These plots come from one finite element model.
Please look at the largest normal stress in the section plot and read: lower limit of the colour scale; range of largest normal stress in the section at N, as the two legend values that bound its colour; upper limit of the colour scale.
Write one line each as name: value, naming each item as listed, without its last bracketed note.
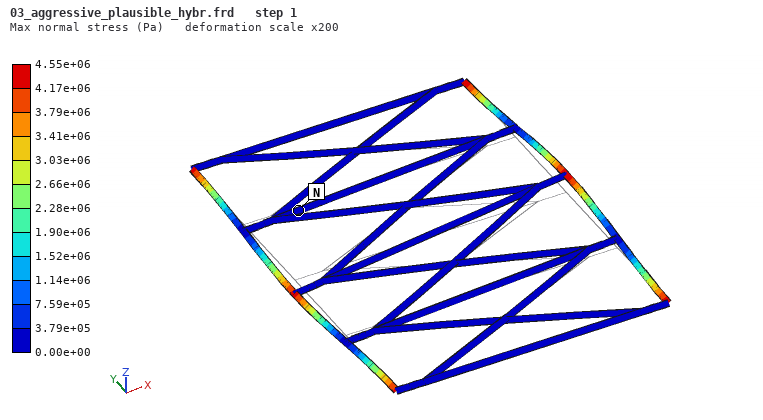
lower limit of the colour scale: 0.00e+00 Pa
range of largest normal stress in the section at N, as the two legend values that bound its colour: 0.00e+00 to 3.79e+05 Pa
upper limit of the colour scale: 4.55e+06 Pa
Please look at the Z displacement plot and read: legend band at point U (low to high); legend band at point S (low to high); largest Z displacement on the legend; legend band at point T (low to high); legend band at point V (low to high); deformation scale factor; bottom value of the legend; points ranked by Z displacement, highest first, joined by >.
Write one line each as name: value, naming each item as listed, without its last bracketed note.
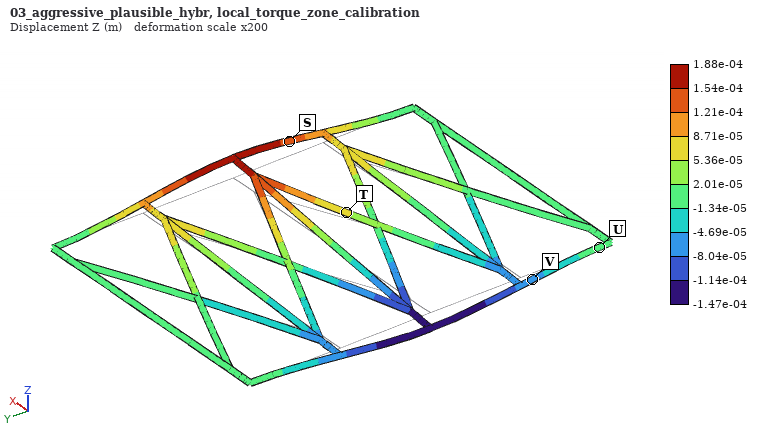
legend band at point U: -1.34e-05 to 2.01e-05 m
legend band at point S: 1.21e-04 to 1.54e-04 m
largest Z displacement on the legend: 1.88e-04 m
legend band at point T: 5.36e-05 to 8.71e-05 m
legend band at point V: -8.04e-05 to -4.69e-05 m
deformation scale factor: 200
bottom value of the legend: -1.47e-04 m
points ranked by Z displacement, highest first, joined by >: S > T > U > V
